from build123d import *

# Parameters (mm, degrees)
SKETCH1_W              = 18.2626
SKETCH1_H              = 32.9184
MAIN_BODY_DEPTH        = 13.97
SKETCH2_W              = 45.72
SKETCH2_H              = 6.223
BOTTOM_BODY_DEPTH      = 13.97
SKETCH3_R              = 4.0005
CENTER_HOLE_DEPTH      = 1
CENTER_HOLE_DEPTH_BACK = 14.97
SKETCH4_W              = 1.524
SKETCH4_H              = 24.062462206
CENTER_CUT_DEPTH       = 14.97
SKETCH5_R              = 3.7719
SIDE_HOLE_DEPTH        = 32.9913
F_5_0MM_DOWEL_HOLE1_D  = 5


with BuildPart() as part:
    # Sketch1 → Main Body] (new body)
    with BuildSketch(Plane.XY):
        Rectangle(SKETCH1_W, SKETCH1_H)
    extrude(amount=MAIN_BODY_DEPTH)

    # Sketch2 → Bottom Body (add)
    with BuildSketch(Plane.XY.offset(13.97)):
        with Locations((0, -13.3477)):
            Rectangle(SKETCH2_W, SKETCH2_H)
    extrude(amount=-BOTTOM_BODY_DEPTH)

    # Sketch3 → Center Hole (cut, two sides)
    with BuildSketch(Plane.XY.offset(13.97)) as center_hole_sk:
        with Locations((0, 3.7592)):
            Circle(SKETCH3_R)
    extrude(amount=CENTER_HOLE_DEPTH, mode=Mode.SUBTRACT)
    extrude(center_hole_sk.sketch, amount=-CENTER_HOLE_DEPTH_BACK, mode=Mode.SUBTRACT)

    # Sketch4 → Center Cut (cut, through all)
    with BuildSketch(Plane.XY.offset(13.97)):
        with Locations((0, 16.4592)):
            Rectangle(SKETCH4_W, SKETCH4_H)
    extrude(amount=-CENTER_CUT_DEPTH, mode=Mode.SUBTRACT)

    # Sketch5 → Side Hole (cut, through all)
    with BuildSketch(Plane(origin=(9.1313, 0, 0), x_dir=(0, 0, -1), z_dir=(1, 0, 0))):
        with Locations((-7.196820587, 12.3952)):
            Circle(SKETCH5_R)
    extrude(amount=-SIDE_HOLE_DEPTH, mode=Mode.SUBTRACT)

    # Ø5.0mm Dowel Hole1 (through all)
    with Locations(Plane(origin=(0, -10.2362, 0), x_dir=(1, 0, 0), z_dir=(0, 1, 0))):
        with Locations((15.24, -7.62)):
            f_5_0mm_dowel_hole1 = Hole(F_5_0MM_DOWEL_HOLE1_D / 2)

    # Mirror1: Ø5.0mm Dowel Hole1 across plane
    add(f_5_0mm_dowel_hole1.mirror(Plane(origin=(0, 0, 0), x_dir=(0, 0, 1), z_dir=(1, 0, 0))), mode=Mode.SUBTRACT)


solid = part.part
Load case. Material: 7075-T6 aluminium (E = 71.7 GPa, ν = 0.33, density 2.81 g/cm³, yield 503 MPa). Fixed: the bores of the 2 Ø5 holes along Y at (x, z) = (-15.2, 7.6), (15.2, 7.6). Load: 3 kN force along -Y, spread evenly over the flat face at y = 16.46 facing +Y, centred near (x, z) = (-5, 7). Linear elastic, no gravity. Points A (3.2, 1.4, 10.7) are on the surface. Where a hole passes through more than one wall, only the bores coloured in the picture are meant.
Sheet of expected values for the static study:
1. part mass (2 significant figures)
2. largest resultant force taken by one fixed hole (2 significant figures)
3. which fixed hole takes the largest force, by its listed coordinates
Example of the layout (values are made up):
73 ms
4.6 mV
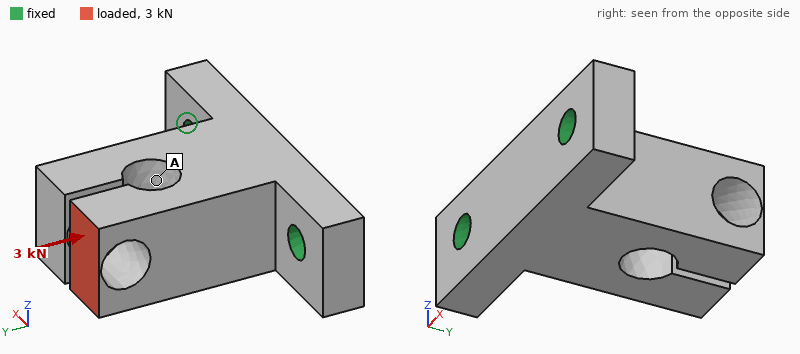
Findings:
25 g
2.2 kN
(-15.2, 7.6)
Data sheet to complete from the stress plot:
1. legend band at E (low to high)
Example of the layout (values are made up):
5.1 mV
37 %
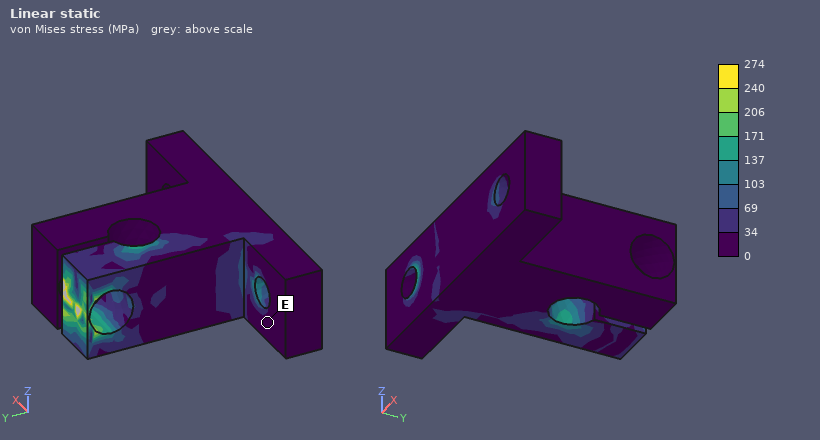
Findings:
0 to 34 MPa
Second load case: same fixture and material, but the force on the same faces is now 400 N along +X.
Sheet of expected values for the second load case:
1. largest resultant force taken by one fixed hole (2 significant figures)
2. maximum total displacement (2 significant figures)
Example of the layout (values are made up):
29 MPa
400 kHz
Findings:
580 N
81 µm
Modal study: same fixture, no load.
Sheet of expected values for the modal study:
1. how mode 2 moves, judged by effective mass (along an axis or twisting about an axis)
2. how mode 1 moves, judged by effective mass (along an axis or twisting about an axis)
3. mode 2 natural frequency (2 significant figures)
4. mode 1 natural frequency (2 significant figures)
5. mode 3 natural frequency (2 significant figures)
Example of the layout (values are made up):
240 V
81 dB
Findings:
along X
along Z
10000 Hz
6000 Hz
12 kHz
